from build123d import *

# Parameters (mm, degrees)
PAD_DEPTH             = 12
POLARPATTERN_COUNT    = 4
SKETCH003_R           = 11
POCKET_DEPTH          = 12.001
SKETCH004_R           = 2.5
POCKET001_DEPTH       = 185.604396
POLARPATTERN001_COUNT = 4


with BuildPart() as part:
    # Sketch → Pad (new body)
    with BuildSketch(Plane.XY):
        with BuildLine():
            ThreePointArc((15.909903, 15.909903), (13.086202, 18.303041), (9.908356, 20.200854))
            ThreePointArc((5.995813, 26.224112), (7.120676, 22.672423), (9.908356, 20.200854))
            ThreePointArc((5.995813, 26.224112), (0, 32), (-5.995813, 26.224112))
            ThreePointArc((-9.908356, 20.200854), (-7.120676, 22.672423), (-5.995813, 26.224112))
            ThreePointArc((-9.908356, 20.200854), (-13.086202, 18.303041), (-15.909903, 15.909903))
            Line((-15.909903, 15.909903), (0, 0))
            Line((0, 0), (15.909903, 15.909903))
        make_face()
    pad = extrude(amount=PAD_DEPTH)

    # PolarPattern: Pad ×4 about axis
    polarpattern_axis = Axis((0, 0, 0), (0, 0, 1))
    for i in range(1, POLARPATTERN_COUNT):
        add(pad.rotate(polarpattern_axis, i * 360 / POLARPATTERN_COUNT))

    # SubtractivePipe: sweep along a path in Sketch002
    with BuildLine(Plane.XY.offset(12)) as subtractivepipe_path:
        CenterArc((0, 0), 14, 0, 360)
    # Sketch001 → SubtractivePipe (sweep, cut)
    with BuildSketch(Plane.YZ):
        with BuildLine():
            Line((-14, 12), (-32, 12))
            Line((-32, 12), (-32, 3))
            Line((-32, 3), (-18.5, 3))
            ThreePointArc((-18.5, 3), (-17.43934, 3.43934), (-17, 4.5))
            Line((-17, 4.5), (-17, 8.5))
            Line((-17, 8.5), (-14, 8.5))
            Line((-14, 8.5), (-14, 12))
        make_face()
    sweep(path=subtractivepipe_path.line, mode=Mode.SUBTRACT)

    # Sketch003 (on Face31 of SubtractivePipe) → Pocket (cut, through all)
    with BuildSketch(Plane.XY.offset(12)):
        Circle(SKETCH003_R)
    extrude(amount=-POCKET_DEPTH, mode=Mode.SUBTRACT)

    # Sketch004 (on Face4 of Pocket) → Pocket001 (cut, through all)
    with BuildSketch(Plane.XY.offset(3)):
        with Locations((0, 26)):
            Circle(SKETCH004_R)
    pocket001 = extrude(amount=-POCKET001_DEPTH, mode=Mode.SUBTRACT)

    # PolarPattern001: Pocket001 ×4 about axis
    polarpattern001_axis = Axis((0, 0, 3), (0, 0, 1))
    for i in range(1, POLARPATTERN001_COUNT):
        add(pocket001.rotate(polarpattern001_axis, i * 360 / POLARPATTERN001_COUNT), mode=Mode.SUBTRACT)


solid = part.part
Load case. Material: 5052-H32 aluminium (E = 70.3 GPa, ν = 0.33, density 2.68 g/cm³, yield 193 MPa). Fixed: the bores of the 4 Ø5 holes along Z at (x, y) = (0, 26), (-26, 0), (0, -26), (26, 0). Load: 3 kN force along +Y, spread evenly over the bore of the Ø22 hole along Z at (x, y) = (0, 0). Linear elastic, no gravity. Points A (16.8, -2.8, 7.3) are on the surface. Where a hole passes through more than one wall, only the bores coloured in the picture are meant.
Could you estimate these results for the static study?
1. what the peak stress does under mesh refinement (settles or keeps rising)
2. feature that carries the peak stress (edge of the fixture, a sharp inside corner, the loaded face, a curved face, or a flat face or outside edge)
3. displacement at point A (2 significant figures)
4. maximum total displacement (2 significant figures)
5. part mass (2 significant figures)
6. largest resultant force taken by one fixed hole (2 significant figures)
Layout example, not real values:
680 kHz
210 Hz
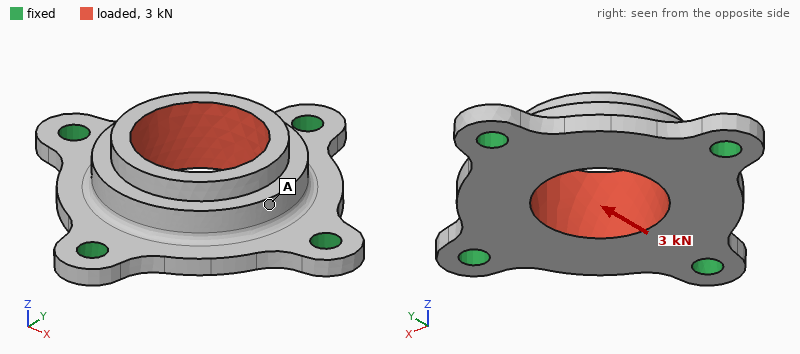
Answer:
keeps rising
edge of the fixture
7.0 µm
12 µm
23 g
1.1 kN
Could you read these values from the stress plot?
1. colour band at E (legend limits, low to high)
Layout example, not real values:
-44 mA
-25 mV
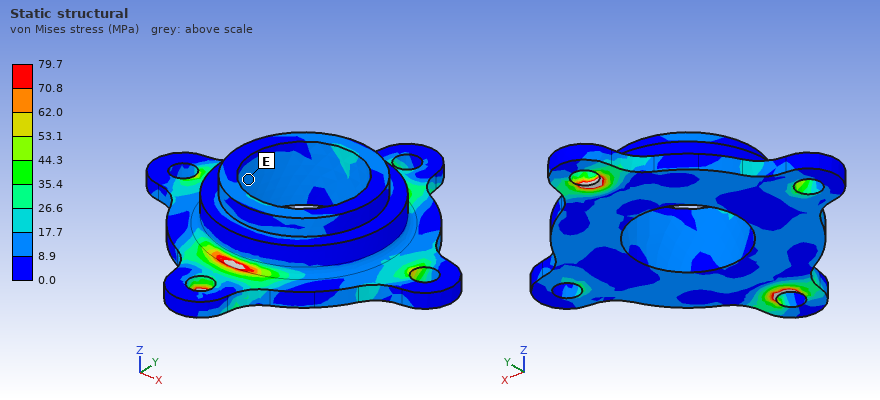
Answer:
8.9 to 17.7 MPa
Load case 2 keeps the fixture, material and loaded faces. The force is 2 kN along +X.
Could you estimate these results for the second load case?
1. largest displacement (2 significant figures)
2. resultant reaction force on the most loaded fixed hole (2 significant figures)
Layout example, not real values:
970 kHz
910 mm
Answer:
8.0 µm
730 N
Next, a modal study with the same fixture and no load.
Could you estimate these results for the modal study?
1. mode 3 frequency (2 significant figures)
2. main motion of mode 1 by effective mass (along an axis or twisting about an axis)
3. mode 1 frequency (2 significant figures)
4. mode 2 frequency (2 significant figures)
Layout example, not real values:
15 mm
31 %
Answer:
15 kHz
along Z
12 kHz
15 kHz
